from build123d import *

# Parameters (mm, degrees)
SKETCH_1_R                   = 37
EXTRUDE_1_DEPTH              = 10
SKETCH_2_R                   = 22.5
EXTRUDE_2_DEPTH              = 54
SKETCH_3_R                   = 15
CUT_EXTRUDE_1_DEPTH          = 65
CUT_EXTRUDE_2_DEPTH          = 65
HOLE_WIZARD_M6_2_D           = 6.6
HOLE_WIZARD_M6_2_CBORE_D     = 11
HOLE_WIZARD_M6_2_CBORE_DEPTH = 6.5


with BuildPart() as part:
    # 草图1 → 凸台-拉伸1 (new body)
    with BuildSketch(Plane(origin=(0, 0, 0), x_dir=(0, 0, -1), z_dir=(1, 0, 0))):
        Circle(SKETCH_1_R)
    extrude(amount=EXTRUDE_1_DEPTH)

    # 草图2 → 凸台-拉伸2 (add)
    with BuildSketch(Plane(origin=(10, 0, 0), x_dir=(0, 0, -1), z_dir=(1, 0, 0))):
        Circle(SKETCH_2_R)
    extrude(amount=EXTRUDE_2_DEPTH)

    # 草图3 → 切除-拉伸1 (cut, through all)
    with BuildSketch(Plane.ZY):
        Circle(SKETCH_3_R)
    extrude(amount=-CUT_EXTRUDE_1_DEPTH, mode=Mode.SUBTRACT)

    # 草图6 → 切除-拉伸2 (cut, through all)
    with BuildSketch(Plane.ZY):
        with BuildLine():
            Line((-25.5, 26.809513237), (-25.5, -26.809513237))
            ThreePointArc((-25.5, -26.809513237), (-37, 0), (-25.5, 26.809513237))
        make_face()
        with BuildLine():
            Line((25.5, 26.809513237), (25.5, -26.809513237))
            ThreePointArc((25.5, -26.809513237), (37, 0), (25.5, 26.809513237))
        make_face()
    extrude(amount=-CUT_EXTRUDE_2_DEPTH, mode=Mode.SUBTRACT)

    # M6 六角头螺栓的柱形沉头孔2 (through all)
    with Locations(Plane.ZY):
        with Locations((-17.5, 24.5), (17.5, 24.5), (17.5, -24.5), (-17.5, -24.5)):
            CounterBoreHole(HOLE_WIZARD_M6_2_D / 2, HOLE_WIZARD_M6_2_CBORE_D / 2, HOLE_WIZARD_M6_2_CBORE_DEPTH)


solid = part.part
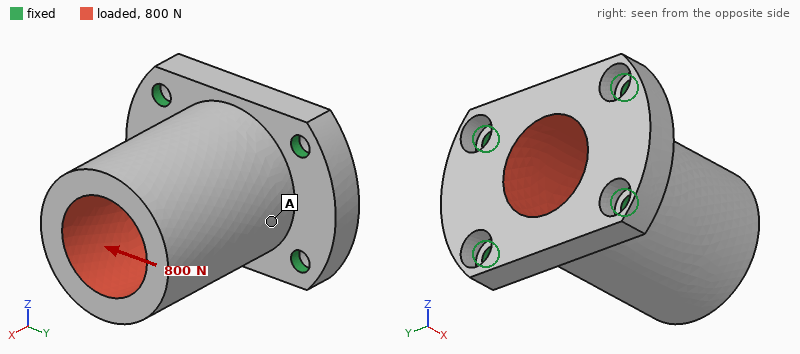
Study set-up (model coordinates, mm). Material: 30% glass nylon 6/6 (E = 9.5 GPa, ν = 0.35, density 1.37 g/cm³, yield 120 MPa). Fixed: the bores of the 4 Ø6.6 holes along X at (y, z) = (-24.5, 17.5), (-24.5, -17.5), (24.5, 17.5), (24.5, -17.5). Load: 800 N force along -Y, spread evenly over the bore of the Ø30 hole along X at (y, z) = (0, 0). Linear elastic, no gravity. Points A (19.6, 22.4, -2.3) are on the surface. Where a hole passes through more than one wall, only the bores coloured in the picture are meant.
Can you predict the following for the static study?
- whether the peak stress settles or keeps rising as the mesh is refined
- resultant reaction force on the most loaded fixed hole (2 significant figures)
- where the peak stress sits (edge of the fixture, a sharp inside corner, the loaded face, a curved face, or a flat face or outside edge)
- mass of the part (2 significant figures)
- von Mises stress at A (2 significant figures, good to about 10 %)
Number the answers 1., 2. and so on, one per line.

1. keeps rising
2. 290 N
3. edge of the fixture
4. 99 g
5. 1.8 MPa
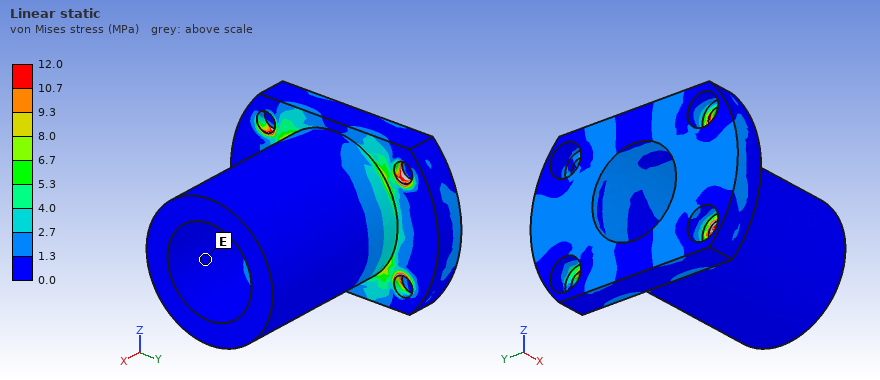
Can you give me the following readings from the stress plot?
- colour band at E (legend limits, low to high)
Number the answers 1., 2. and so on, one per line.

1. 0.0 to 1.3 MPa
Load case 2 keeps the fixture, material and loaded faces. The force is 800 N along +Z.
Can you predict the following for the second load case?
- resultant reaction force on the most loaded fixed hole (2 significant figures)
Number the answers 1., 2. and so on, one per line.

1. 340 N
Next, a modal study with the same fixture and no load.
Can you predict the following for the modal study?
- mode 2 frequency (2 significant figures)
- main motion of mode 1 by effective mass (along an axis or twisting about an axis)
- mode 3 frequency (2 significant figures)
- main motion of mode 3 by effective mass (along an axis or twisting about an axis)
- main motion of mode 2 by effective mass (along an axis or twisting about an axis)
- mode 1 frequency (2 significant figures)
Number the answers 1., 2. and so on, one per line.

1. 2700 Hz
2. along Z
3. 4500 Hz
4. along X
5. along Y
6. 2100 Hz
